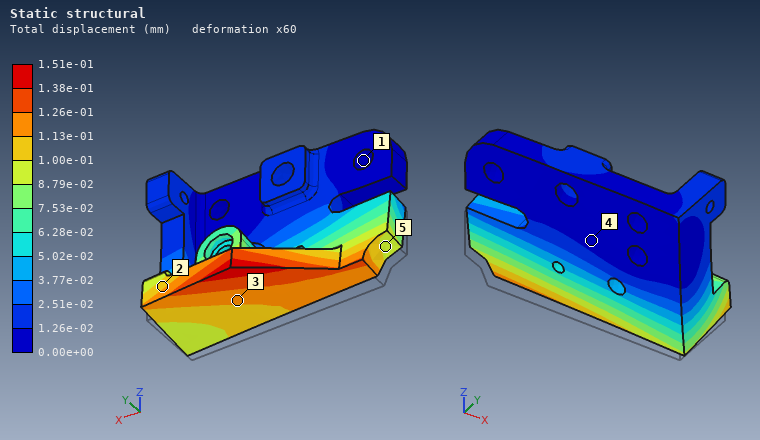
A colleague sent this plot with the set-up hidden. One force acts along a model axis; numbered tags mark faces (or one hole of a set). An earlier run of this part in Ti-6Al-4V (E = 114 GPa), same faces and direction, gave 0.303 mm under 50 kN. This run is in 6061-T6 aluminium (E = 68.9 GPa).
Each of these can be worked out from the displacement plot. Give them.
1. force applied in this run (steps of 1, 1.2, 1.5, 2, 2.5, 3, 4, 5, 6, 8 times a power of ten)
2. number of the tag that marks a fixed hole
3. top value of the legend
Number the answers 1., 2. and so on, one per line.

1. 15 kN
2. 1
3. 1.51e-01 mm
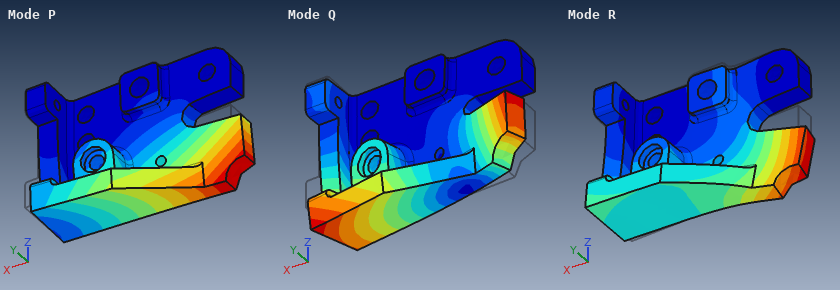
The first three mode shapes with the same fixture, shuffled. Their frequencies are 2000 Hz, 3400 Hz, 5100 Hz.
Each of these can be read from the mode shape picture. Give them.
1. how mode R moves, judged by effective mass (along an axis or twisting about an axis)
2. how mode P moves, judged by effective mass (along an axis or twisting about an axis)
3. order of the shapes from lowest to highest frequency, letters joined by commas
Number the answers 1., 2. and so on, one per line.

1. along X
2. along Y
3. P, Q, R
